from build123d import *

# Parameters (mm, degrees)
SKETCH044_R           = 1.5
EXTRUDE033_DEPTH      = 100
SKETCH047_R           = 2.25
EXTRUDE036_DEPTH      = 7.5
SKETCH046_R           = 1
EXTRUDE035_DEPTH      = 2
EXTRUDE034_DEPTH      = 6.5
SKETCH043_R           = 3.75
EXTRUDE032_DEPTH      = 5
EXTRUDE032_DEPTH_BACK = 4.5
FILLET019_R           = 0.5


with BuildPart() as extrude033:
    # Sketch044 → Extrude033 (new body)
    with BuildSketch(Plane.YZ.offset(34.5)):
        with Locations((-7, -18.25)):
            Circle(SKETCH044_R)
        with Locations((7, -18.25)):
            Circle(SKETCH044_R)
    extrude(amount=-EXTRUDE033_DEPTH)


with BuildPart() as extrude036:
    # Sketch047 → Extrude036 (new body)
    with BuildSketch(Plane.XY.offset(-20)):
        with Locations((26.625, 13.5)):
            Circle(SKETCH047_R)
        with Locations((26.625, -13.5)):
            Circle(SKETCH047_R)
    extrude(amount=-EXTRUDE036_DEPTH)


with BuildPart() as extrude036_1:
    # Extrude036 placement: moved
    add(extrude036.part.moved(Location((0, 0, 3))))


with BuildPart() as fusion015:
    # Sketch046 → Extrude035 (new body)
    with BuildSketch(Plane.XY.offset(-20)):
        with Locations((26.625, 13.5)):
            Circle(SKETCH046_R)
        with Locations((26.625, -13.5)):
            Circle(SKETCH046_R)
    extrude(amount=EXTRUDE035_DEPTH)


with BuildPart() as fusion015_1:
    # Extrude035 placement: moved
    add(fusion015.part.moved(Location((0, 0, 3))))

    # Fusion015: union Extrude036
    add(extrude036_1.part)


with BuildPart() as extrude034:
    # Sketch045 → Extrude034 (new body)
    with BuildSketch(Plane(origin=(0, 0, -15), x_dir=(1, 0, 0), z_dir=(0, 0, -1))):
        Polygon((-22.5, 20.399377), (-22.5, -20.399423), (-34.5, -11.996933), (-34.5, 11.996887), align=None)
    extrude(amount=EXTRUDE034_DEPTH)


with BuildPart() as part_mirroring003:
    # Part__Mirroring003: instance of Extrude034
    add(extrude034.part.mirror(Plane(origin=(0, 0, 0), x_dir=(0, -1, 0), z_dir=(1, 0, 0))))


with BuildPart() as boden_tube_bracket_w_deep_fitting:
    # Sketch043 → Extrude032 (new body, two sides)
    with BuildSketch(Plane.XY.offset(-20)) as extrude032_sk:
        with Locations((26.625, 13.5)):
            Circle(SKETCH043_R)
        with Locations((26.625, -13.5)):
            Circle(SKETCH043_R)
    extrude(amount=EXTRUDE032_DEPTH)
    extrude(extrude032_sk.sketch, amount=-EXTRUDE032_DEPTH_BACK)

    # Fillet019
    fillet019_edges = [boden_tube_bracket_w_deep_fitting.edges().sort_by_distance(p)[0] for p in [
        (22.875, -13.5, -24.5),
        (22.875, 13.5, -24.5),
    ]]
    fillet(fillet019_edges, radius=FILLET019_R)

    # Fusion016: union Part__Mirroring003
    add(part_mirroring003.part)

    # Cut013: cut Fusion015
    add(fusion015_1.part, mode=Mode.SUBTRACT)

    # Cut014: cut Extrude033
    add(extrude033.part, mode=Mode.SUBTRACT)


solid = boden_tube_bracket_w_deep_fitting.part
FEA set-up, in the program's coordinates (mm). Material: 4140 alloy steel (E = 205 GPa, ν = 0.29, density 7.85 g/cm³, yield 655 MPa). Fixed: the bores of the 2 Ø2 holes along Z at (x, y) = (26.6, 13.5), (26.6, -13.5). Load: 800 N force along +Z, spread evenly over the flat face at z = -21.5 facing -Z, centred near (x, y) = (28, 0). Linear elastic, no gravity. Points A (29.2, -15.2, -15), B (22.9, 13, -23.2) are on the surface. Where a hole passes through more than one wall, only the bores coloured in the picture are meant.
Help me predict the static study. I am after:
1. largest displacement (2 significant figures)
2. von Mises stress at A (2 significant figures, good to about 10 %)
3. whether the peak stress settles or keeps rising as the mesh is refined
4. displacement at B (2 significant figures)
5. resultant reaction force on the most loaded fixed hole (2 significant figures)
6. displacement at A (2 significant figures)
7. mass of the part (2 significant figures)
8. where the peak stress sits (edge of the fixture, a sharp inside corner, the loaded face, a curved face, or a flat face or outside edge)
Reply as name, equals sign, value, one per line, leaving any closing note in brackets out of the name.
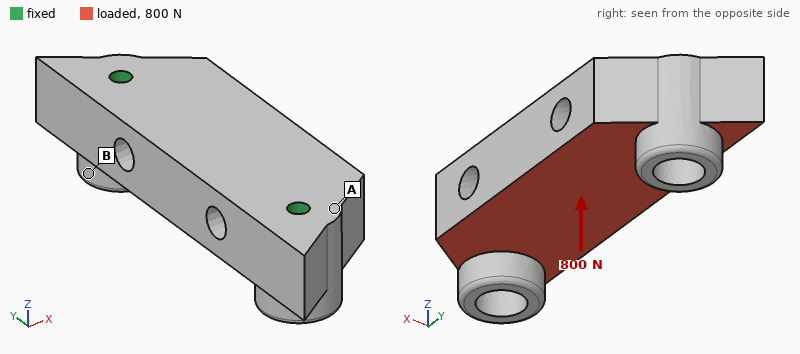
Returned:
largest displacement = 8.5 µm
von Mises stress at A = 28 MPa
whether the peak stress settles or keeps rising as the mesh is refined = keeps rising
displacement at B = 3.8 µm
resultant reaction force on the most loaded fixed hole = 470 N
displacement at A = 1.5 µm
mass of the part = 19 g
where the peak stress sits = edge of the fixture
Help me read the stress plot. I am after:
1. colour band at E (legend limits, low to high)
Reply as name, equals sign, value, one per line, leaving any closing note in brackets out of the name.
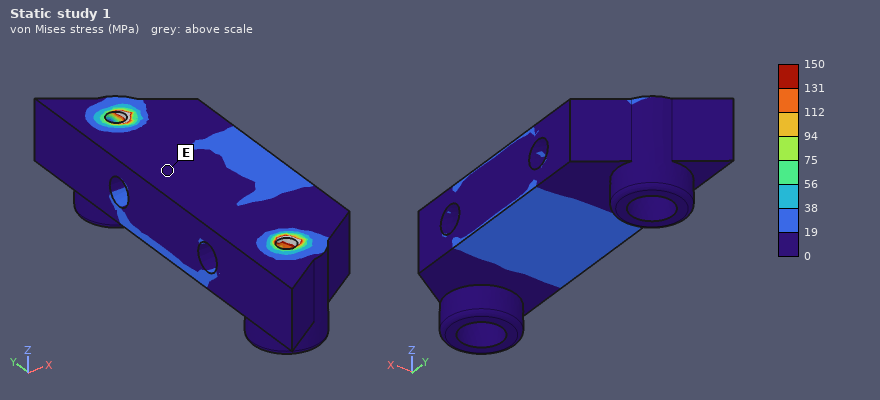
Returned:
colour band at E = 0 to 19 MPa
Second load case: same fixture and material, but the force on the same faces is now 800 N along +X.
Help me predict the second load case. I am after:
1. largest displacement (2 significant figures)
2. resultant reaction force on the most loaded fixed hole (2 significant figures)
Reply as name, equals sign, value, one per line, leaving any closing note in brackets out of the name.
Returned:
largest displacement = 18 µm
resultant reaction force on the most loaded fixed hole = 410 N
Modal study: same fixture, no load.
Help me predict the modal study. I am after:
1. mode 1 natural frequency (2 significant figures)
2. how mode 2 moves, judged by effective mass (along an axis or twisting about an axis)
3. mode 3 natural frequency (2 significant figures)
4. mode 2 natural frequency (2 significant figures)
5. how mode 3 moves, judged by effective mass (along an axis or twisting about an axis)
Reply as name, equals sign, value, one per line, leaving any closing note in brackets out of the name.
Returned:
mode 1 natural frequency = 12 kHz
how mode 2 moves, judged by effective mass = along Z
mode 3 natural frequency = 30 kHz
mode 2 natural frequency = 22 kHz
how mode 3 moves, judged by effective mass = along X
